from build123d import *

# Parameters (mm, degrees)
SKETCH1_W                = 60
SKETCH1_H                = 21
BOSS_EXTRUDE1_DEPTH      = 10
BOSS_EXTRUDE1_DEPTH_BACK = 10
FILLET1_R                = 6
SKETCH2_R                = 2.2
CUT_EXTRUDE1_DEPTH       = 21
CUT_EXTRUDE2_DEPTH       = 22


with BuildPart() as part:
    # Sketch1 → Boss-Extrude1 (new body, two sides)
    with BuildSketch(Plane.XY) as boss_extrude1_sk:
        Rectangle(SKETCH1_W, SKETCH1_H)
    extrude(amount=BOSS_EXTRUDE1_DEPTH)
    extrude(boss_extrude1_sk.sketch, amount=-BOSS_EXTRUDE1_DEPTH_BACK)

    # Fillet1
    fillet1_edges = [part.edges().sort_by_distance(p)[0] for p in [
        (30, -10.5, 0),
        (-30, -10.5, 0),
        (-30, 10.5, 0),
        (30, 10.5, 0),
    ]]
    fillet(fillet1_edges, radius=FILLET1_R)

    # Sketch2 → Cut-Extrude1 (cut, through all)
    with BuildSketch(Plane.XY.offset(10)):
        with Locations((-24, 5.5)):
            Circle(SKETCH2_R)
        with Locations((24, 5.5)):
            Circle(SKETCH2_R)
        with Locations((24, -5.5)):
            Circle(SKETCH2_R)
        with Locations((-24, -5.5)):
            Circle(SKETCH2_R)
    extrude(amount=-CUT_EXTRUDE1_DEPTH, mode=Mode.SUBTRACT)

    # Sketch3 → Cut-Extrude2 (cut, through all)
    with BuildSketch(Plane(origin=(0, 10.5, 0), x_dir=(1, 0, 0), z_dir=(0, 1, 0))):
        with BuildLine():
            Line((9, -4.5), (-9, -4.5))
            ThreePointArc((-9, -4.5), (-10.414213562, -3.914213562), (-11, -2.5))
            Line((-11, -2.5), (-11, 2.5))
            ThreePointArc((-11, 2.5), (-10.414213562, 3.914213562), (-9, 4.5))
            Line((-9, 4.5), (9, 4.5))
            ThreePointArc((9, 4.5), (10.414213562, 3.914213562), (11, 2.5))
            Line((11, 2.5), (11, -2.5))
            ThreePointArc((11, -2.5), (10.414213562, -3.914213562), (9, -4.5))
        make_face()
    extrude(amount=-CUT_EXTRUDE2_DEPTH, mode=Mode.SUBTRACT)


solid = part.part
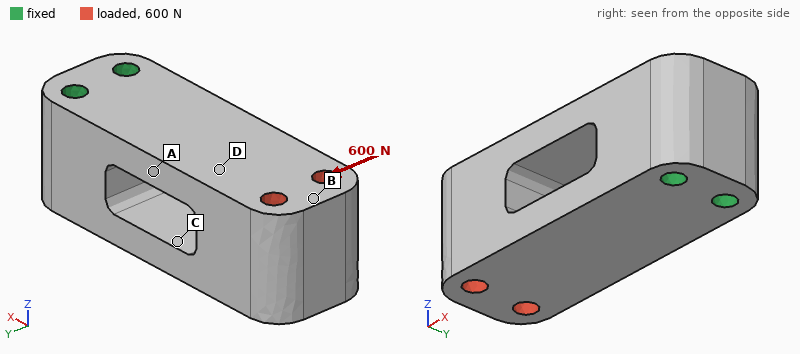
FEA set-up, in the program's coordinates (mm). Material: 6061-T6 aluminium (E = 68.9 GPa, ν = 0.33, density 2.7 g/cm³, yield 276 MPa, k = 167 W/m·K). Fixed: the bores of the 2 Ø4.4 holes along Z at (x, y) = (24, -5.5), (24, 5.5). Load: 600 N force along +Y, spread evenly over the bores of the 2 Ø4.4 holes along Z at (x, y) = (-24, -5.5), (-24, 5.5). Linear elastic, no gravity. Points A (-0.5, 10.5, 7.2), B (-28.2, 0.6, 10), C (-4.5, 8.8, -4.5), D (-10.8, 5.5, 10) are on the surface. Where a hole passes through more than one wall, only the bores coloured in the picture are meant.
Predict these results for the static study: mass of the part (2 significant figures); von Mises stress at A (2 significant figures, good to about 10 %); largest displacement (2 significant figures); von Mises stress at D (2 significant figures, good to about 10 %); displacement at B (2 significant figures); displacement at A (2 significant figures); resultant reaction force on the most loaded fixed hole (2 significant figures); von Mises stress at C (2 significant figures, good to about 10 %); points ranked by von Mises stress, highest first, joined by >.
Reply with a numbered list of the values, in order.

1. 52 g
2. 17 MPa
3. 40 µm
4. 8.3 MPa
5. 38 µm
6. 13 µm
7. 2.1 kN
8. 13 MPa
9. A > C > D > B
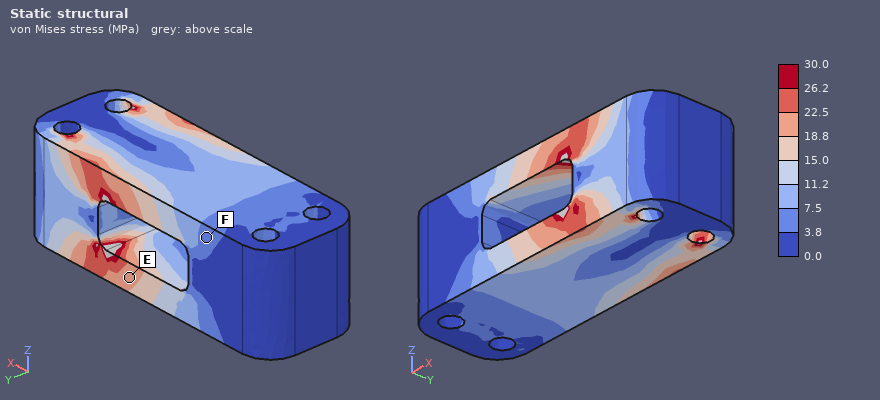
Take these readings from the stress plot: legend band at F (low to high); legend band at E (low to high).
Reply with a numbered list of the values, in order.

1. 3.8 to 7.5 MPa
2. 18.8 to 22.5 MPa
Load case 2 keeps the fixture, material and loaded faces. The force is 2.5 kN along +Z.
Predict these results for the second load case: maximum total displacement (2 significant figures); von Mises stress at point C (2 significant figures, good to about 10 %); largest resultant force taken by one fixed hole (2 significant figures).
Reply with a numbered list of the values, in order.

1. 0.21 mm
2. 75 MPa
3. 1.3 kN
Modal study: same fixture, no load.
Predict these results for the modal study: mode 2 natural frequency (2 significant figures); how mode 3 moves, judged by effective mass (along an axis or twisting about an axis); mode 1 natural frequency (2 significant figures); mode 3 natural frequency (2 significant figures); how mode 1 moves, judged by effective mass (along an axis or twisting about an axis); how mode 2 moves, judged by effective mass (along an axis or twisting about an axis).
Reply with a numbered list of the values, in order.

1. 5000 Hz
2. twisting about X
3. 4000 Hz
4. 10 kHz
5. along Z
6. along Y
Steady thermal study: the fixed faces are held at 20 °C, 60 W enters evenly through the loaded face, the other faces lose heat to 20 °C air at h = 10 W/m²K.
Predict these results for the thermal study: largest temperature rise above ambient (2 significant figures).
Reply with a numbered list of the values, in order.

1. 59 K
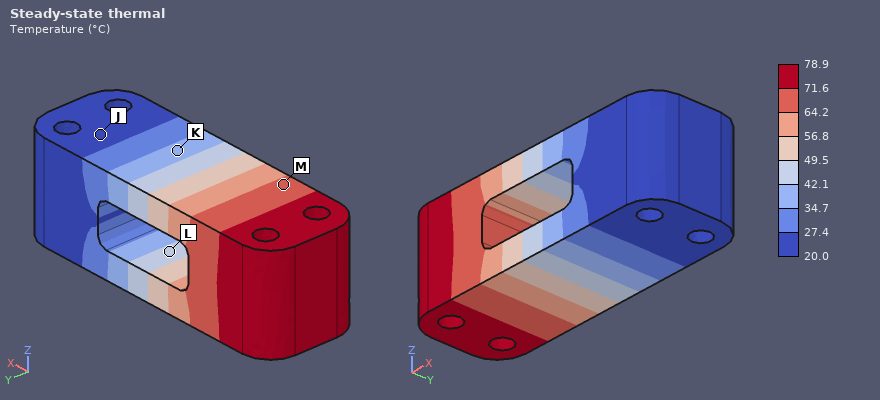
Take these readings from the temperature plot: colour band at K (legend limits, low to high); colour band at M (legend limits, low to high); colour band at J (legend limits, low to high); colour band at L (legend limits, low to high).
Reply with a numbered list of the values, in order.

1. 34.7 to 42.1 °C
2. 64.2 to 71.6 °C
3. 20.0 to 27.4 °C
4. 42.1 to 49.5 °C
